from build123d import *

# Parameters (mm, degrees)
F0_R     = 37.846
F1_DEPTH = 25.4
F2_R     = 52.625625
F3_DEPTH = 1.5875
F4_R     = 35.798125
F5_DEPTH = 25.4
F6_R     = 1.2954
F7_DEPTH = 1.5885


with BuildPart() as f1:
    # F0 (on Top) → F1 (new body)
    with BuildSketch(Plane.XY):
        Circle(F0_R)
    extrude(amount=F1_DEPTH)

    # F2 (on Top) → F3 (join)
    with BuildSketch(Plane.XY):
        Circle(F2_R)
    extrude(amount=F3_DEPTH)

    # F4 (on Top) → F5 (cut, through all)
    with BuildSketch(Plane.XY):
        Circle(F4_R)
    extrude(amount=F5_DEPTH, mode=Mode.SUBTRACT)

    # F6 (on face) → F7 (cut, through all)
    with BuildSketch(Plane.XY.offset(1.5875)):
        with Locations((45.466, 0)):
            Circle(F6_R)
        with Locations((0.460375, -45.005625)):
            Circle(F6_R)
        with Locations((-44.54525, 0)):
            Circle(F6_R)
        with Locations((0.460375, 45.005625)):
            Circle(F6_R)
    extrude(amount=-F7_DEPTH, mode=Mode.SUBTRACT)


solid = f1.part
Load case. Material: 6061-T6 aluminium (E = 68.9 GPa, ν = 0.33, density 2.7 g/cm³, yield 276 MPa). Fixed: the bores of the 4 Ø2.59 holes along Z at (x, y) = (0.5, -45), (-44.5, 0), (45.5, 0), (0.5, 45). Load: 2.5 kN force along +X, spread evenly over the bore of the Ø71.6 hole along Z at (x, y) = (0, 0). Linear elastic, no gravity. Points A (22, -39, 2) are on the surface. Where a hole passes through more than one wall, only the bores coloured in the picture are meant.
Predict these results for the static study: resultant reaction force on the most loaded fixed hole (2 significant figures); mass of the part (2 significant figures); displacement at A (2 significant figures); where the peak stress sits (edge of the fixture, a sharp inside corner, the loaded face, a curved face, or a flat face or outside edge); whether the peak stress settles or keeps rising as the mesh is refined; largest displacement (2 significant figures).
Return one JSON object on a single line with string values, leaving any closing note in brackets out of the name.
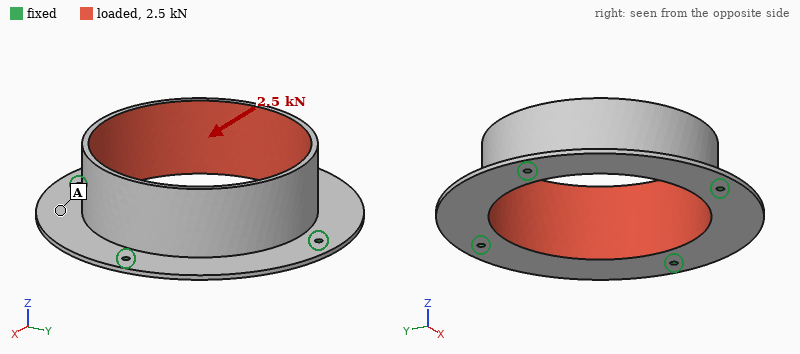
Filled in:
{"resultant reaction force on the most loaded fixed hole": "800 N", "mass of the part": "50 g", "displacement at A": "0.061 mm", "where the peak stress sits": "edge of the fixture", "whether the peak stress settles or keeps rising as the mesh is refined": "keeps rising", "largest displacement": "0.11 mm"}
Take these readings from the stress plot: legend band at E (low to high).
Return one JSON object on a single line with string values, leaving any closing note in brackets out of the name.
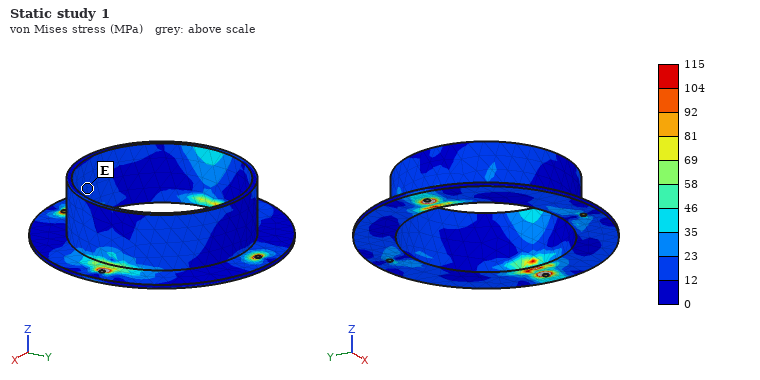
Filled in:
{"legend band at E": "12 to 23 MPa"}
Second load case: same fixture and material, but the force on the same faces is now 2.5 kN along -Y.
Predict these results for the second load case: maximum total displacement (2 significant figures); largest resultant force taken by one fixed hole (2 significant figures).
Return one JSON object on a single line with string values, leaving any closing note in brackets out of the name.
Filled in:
{"maximum total displacement": "0.11 mm", "largest resultant force taken by one fixed hole": "810 N"}
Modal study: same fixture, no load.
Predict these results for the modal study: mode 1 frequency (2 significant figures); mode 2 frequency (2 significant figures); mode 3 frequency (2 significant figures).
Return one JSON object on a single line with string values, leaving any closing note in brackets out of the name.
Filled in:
{"mode 1 frequency": "1700 Hz", "mode 2 frequency": "2600 Hz", "mode 3 frequency": "2600 Hz"}
